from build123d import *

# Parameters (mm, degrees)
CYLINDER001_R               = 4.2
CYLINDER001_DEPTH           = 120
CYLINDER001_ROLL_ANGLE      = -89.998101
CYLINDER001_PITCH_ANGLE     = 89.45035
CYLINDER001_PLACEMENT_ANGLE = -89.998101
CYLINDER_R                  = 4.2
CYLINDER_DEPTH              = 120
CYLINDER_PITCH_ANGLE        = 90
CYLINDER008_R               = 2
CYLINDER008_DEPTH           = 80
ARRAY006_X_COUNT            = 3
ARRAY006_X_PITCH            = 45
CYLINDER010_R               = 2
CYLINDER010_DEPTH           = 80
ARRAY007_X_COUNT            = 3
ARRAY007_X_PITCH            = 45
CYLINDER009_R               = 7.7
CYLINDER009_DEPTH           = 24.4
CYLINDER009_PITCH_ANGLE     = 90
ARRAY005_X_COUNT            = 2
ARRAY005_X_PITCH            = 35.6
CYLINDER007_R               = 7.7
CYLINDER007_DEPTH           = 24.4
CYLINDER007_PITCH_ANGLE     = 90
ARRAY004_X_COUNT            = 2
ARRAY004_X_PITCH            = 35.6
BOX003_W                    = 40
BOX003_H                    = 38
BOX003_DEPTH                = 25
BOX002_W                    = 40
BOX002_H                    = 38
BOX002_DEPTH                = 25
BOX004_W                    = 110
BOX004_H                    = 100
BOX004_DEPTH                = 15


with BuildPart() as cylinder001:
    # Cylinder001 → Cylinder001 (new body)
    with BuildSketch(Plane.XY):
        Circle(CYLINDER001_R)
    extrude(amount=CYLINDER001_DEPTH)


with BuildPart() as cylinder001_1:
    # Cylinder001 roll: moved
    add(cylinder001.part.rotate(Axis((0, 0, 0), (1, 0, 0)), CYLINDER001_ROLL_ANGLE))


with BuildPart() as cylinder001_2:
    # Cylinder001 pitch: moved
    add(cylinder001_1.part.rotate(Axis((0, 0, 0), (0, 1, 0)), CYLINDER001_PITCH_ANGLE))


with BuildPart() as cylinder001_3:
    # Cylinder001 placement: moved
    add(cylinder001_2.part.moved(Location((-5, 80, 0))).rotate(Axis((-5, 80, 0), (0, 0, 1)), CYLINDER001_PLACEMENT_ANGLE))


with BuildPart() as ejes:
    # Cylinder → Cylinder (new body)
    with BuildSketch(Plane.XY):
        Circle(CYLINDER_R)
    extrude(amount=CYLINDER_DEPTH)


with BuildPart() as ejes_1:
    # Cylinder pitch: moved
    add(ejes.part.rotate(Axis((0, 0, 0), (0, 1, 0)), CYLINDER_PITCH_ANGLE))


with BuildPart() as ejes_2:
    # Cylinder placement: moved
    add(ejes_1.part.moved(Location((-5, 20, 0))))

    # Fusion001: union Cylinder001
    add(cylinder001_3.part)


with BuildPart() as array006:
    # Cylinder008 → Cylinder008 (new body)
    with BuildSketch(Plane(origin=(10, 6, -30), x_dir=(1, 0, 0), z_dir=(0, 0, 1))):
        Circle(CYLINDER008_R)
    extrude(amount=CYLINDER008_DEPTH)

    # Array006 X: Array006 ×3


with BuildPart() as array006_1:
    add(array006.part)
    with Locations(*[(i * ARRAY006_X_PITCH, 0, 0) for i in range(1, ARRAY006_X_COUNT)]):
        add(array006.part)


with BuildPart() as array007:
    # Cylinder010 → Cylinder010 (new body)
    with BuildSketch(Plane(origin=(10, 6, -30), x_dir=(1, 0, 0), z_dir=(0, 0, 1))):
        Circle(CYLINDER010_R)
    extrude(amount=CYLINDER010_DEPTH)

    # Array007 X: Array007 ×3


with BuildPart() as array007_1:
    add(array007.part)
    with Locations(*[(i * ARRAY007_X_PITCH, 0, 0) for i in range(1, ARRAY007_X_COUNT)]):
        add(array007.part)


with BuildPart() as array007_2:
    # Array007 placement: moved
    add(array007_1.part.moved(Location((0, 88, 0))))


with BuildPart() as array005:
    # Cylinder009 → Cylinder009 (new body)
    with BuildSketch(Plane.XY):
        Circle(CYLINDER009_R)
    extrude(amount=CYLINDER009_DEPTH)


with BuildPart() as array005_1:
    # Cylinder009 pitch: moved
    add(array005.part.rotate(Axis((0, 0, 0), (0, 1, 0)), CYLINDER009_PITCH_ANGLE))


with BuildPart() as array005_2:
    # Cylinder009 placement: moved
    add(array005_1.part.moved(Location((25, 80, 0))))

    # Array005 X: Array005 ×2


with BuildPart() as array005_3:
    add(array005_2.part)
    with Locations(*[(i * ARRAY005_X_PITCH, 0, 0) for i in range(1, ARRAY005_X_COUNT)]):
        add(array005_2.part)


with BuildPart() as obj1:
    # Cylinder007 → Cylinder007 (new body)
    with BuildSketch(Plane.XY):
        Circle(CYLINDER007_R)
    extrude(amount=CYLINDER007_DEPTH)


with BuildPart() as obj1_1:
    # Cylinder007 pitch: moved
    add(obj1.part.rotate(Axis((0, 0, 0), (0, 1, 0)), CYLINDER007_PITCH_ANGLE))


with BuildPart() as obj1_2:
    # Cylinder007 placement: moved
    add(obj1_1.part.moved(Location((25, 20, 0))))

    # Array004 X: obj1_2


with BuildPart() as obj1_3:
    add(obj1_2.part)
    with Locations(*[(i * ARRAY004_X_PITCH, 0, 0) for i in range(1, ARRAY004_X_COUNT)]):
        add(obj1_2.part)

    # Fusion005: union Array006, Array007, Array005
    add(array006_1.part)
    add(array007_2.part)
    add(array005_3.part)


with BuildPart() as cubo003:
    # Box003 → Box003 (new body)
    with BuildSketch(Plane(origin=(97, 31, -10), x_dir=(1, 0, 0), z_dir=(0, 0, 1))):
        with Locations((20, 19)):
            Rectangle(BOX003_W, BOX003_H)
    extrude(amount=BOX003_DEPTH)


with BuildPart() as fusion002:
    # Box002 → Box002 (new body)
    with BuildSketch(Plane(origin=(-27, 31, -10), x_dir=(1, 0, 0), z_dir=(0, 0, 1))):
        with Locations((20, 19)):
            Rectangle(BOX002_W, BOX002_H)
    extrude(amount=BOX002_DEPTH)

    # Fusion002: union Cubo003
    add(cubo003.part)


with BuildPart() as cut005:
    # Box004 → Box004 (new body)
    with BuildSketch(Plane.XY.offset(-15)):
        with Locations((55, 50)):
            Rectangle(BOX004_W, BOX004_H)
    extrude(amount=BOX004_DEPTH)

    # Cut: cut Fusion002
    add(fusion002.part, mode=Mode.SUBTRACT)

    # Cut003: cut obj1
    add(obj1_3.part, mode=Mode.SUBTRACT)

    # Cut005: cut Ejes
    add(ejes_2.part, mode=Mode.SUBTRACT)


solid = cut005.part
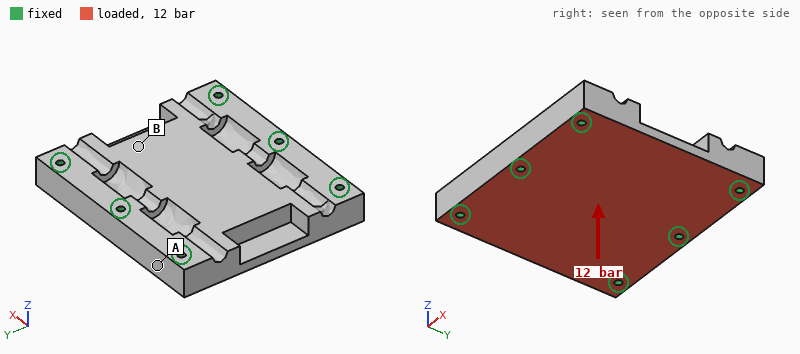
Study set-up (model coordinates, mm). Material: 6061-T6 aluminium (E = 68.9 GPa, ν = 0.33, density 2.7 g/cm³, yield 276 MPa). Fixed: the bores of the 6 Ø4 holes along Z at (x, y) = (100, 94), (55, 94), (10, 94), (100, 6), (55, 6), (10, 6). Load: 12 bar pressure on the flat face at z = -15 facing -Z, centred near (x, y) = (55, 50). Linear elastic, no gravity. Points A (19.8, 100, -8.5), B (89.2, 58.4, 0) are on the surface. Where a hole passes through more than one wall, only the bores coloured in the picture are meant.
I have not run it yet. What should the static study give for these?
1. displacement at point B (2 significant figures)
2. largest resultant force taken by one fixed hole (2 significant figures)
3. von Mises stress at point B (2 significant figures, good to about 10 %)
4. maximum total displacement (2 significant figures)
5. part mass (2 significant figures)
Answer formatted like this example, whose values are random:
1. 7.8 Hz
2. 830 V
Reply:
1. 23 µm
2. 2.6 kN
3. 16 MPa
4. 32 µm
5. 380 g
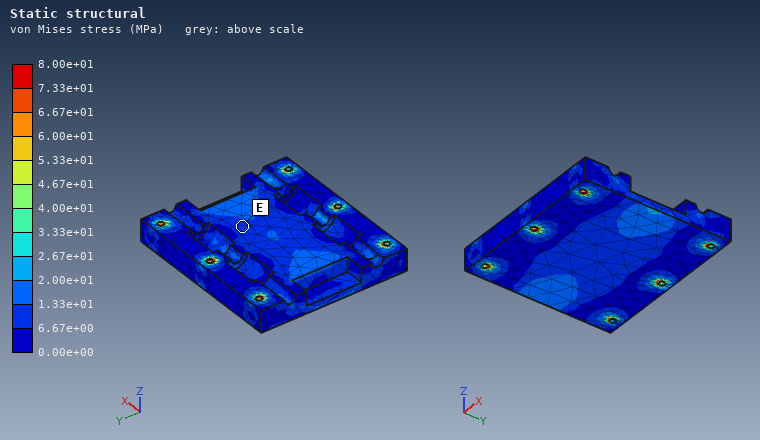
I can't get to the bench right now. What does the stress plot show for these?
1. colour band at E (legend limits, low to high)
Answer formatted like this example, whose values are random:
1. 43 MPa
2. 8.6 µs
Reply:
1. 6.67e+00 to 1.33e+01 MPa
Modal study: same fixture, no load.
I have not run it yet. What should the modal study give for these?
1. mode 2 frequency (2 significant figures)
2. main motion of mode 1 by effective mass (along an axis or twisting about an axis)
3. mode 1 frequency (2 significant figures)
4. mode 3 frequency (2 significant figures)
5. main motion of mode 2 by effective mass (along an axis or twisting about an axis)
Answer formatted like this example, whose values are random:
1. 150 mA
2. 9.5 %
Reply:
1. 8400 Hz
2. along Z
3. 6800 Hz
4. 13 kHz
5. twisting about Y
